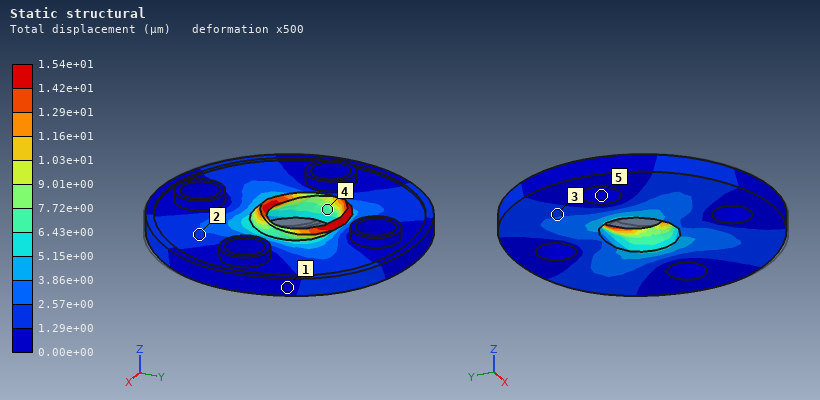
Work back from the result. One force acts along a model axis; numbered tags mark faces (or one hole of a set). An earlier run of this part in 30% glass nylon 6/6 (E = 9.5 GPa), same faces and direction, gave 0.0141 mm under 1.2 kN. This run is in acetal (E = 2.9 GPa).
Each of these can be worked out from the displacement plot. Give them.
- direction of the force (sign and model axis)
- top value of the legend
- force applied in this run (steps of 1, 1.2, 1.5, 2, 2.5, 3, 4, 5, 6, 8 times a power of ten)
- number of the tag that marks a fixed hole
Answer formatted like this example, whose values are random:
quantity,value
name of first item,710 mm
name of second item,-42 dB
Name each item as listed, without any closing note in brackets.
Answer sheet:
quantity,value
direction of the force,+Y
top value of the legend,1.54e+01 µm
force applied in this run,400 N
number of the tag that marks a fixed hole,5
